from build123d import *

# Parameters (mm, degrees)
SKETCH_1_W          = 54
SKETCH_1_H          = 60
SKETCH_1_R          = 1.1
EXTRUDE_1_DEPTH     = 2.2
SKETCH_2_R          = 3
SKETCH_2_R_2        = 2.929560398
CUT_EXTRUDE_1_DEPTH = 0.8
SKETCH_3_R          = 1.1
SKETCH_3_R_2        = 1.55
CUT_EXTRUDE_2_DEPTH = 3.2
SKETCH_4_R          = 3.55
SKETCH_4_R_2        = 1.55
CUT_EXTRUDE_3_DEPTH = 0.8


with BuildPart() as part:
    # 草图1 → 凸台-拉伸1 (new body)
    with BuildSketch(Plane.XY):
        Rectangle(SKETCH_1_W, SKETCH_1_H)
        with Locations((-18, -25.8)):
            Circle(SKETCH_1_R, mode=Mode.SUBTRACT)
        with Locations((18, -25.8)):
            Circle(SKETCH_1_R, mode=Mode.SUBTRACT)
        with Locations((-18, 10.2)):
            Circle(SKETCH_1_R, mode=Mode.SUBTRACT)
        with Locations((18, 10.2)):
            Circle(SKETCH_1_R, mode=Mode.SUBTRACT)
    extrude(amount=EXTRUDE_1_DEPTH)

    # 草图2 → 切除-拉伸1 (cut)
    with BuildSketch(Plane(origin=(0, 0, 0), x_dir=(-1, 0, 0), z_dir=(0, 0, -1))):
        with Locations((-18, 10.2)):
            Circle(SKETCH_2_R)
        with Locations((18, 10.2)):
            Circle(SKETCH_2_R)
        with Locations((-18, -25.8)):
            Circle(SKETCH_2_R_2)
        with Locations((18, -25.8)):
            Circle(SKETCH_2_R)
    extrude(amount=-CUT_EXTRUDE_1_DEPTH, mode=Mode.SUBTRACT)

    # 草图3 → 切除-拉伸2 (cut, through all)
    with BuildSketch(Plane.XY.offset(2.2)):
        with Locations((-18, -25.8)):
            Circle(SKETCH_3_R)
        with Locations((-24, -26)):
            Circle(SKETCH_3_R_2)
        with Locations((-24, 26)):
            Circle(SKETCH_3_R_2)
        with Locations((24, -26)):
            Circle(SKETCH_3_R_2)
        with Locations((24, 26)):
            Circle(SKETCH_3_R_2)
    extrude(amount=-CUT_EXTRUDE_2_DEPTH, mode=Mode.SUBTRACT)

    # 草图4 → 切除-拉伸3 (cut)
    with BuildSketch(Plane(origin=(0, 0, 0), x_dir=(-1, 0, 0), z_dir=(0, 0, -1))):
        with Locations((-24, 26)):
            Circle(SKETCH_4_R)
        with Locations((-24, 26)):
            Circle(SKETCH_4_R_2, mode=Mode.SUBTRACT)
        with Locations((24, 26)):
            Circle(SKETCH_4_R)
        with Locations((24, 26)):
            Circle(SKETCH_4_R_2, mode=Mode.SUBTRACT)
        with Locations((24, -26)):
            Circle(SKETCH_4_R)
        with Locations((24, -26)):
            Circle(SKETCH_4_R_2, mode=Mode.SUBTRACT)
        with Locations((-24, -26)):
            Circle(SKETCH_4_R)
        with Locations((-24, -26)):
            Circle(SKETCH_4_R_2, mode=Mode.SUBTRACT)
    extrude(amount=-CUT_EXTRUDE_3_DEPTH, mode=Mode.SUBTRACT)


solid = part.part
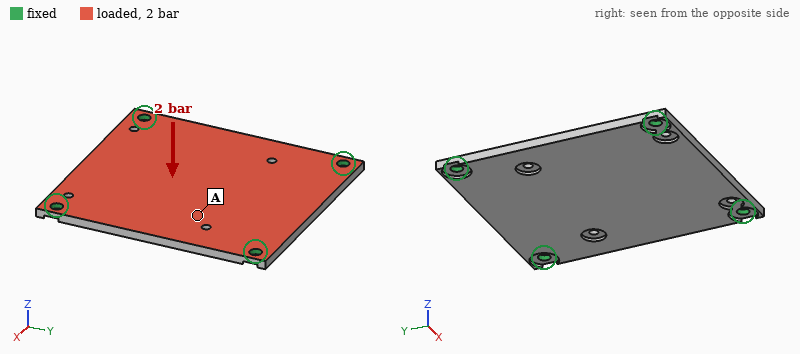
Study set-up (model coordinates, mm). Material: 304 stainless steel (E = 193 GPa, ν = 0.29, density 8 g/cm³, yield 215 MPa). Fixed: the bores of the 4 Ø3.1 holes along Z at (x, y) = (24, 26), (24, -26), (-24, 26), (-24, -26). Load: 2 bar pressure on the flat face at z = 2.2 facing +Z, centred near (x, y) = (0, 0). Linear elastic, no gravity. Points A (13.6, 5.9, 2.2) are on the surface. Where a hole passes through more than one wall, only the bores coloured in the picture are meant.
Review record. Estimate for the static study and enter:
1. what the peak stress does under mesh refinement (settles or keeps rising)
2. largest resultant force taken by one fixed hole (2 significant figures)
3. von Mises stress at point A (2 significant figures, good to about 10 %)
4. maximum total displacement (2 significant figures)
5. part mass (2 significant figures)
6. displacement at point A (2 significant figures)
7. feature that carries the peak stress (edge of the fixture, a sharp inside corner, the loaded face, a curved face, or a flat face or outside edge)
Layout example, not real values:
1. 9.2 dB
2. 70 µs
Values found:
1. keeps rising
2. 310 N
3. 32 MPa
4. 70 µm
5. 55 g
6. 58 µm
7. edge of the fixture
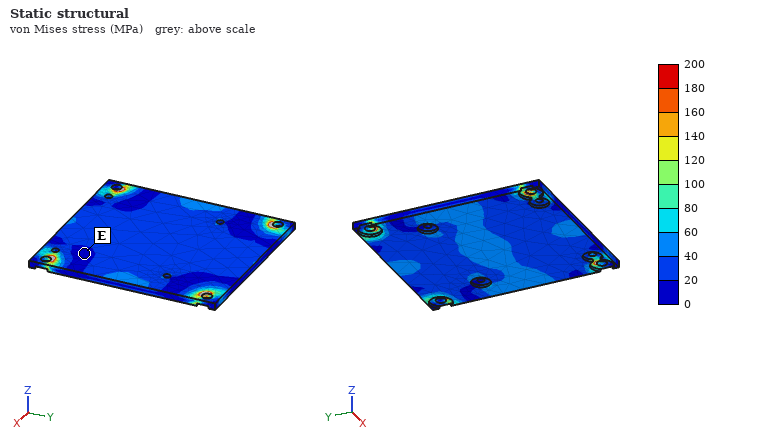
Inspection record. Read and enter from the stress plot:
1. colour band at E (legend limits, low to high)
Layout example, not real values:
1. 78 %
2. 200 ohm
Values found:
1. 0 to 20 MPa
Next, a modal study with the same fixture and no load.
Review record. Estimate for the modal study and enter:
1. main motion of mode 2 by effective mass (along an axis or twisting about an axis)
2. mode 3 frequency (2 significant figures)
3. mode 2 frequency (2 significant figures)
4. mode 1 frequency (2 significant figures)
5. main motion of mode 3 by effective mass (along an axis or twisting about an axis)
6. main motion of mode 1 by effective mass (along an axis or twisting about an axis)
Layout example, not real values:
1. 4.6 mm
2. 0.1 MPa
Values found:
1. twisting about Y
2. 4500 Hz
3. 4200 Hz
4. 2400 Hz
5. twisting about X
6. along Z
